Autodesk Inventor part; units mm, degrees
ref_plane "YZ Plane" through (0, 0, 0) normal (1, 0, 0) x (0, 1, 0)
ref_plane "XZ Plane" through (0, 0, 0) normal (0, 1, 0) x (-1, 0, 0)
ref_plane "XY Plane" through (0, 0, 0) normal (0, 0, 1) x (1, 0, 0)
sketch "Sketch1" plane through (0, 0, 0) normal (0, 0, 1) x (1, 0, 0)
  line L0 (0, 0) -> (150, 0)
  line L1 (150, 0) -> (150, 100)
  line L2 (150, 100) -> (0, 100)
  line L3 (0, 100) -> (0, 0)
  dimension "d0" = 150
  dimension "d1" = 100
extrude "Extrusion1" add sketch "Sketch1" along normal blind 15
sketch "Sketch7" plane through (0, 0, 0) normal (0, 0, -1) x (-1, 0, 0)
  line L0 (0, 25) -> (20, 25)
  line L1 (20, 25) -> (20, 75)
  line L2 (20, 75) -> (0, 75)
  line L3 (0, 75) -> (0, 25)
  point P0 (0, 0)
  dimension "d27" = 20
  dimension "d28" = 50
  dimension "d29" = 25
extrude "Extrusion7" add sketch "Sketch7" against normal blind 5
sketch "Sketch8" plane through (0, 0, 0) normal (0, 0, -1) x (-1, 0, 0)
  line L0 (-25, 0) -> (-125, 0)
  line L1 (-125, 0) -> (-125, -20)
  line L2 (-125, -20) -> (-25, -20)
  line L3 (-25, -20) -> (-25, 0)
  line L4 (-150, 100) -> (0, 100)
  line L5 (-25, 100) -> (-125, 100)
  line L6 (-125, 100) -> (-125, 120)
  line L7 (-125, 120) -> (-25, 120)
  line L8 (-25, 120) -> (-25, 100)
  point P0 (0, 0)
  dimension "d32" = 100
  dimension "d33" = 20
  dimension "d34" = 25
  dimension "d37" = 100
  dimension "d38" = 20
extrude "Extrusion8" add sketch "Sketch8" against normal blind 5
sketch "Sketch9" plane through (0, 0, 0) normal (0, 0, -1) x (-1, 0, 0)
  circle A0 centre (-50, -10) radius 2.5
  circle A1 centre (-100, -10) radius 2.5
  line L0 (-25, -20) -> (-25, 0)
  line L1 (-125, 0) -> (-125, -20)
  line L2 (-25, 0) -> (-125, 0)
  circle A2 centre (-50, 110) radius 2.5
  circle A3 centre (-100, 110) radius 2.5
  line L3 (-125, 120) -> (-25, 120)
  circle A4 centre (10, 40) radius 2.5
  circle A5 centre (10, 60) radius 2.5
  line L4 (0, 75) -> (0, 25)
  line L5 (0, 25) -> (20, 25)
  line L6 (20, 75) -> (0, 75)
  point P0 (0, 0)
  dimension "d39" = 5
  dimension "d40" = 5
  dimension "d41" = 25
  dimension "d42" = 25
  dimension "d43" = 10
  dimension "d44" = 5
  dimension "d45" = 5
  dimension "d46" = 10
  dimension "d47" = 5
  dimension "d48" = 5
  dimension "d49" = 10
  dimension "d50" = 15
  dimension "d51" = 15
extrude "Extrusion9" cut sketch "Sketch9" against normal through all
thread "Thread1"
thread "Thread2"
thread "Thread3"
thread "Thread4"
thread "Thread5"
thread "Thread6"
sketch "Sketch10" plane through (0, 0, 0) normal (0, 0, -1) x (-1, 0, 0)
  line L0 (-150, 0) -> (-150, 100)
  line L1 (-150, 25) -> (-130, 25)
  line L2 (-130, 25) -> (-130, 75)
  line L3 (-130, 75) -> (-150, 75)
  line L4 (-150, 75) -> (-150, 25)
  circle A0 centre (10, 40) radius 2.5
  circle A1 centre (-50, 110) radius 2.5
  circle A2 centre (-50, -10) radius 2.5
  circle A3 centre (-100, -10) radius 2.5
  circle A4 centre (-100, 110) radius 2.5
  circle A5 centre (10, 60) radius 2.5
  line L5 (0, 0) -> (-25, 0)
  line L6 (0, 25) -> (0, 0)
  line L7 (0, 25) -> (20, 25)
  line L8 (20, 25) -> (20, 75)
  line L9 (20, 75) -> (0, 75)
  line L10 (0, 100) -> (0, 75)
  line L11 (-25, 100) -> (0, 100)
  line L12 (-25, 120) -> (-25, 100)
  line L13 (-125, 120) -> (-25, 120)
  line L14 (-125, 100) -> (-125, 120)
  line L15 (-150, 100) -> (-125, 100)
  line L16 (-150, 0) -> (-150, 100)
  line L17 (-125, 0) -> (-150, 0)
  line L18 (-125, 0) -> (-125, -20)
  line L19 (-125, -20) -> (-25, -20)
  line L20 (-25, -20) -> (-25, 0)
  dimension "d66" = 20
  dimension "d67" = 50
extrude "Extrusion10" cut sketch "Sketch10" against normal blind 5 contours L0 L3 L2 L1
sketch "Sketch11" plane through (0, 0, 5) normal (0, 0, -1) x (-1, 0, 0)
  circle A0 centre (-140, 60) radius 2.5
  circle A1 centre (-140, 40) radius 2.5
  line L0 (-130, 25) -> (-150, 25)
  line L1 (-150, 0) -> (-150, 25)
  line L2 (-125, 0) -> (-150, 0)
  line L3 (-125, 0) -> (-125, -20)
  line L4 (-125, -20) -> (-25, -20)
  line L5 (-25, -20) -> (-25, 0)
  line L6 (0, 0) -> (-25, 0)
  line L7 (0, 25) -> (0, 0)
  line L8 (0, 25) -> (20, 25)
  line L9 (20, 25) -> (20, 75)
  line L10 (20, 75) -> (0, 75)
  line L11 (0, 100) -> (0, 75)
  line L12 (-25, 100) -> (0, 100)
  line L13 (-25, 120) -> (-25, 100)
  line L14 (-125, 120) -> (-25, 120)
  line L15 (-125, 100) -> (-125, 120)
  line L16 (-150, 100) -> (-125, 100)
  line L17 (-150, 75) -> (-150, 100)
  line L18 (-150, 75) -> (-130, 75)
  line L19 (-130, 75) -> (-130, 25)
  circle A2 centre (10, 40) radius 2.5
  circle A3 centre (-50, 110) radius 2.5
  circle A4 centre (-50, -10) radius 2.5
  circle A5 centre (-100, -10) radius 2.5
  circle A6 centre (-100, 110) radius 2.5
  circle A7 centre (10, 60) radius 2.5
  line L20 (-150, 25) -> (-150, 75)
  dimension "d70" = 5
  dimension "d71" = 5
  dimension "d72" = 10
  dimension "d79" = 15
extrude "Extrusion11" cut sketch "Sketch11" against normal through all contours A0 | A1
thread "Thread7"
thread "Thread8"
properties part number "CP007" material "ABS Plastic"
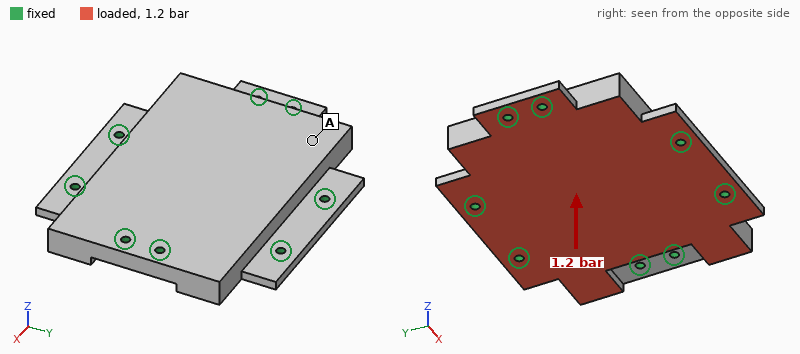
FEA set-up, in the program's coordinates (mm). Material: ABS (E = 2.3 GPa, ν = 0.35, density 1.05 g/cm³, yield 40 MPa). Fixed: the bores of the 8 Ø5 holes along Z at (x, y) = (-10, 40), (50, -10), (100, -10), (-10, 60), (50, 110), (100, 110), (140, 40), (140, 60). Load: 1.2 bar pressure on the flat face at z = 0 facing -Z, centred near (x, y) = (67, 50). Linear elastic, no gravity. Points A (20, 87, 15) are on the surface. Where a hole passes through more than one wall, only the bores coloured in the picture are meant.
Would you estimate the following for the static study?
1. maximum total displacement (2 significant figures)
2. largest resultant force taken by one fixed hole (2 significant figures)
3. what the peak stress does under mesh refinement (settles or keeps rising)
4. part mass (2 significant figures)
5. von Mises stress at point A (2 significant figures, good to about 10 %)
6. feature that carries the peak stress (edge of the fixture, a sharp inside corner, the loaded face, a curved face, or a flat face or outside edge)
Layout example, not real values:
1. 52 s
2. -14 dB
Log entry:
1. 0.22 mm
2. 420 N
3. keeps rising
4. 260 g
5. 2.1 MPa
6. edge of the fixture
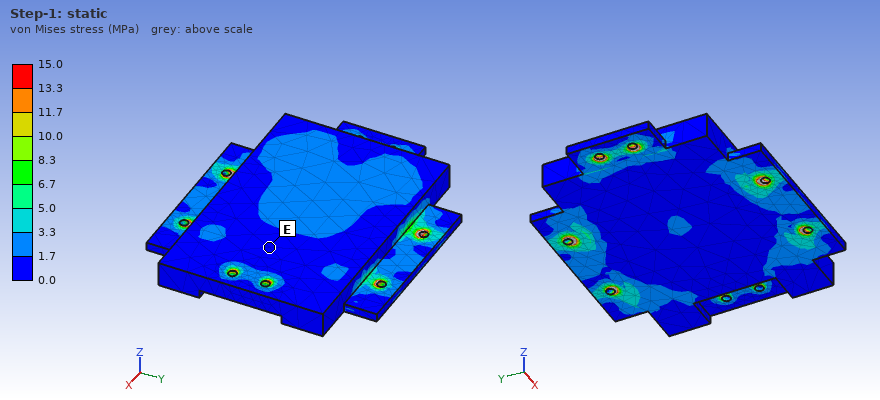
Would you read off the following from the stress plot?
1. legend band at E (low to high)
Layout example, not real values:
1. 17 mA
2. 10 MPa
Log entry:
1. 0.0 to 1.7 MPa
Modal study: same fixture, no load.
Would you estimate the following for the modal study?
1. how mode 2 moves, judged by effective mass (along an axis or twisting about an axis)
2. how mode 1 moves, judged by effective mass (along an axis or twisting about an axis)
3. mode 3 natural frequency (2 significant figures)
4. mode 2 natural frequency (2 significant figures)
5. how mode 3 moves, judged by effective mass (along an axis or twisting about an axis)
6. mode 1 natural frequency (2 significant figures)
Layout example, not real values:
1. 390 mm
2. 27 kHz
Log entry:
1. twisting about X
2. along Z
3. 1700 Hz
4. 1500 Hz
5. twisting about Y
6. 1100 Hz
